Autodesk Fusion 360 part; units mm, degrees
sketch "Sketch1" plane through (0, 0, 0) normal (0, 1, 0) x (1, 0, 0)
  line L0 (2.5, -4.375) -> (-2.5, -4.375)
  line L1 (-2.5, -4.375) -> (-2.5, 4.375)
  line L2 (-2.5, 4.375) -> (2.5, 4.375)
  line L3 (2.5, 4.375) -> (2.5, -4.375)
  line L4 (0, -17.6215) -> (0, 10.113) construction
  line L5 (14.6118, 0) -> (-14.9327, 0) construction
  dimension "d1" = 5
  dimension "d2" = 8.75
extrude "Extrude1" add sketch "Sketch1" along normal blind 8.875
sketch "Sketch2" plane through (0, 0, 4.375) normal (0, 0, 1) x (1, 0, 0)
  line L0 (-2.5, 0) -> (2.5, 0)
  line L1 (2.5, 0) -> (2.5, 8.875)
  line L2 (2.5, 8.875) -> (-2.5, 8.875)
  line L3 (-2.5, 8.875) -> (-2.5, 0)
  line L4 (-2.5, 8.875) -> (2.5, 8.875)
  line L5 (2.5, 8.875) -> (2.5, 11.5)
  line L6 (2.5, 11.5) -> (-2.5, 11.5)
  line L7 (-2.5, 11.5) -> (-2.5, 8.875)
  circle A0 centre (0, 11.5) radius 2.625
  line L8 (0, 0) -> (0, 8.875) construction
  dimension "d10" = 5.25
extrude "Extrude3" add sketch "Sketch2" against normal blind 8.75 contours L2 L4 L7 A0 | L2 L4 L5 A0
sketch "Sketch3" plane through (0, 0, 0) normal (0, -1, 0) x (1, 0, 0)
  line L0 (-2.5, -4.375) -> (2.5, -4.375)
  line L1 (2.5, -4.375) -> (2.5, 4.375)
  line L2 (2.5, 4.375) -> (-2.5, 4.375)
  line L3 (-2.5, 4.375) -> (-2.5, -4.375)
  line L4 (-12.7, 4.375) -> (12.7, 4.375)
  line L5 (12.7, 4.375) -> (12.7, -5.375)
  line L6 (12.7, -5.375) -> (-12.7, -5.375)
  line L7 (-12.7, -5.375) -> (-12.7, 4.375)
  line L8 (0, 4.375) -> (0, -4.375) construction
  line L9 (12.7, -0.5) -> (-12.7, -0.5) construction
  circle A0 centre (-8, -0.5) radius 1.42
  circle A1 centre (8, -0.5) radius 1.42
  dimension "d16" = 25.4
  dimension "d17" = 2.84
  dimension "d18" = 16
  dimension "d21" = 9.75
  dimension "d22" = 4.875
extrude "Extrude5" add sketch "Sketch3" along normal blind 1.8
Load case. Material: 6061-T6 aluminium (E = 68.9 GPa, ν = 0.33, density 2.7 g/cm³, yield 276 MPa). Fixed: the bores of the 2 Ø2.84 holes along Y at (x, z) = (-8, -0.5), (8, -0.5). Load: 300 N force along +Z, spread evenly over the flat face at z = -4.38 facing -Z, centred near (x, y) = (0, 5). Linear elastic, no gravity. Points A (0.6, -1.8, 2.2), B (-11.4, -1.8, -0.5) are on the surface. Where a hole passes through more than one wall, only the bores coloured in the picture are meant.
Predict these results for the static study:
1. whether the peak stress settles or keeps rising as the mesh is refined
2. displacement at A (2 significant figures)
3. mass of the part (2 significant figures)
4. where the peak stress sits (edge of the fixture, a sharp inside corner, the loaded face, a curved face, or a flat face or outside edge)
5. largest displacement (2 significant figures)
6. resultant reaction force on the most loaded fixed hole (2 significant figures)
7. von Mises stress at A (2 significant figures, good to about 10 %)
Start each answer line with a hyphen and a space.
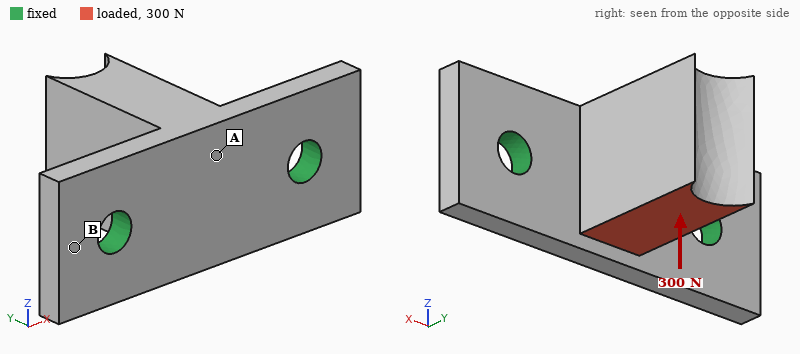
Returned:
- keeps rising
- 18 µm
- 2.2 g
- edge of the fixture
- 91 µm
- 150 N
- 47 MPa
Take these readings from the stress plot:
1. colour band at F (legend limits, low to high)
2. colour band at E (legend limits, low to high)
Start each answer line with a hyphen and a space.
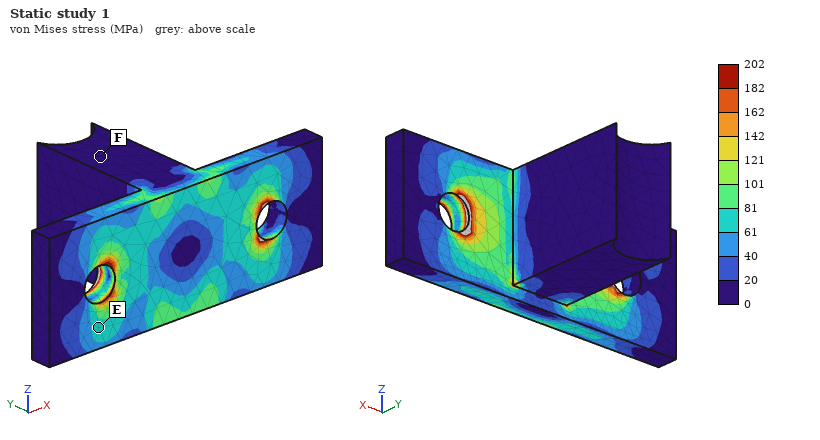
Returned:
- 0 to 20 MPa
- 61 to 81 MPa
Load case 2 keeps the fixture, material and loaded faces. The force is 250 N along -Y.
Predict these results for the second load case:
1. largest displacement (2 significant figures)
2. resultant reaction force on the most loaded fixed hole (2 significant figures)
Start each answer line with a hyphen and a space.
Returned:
- 54 µm
- 130 N
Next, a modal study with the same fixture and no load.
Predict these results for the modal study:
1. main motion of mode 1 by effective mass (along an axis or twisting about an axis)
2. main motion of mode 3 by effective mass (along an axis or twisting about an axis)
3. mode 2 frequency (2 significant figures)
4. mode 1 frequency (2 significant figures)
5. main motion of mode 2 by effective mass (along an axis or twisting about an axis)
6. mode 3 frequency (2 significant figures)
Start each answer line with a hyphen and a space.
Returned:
- along Z
- along Y
- 18 kHz
- 10 kHz
- along X
- 23 kHz
